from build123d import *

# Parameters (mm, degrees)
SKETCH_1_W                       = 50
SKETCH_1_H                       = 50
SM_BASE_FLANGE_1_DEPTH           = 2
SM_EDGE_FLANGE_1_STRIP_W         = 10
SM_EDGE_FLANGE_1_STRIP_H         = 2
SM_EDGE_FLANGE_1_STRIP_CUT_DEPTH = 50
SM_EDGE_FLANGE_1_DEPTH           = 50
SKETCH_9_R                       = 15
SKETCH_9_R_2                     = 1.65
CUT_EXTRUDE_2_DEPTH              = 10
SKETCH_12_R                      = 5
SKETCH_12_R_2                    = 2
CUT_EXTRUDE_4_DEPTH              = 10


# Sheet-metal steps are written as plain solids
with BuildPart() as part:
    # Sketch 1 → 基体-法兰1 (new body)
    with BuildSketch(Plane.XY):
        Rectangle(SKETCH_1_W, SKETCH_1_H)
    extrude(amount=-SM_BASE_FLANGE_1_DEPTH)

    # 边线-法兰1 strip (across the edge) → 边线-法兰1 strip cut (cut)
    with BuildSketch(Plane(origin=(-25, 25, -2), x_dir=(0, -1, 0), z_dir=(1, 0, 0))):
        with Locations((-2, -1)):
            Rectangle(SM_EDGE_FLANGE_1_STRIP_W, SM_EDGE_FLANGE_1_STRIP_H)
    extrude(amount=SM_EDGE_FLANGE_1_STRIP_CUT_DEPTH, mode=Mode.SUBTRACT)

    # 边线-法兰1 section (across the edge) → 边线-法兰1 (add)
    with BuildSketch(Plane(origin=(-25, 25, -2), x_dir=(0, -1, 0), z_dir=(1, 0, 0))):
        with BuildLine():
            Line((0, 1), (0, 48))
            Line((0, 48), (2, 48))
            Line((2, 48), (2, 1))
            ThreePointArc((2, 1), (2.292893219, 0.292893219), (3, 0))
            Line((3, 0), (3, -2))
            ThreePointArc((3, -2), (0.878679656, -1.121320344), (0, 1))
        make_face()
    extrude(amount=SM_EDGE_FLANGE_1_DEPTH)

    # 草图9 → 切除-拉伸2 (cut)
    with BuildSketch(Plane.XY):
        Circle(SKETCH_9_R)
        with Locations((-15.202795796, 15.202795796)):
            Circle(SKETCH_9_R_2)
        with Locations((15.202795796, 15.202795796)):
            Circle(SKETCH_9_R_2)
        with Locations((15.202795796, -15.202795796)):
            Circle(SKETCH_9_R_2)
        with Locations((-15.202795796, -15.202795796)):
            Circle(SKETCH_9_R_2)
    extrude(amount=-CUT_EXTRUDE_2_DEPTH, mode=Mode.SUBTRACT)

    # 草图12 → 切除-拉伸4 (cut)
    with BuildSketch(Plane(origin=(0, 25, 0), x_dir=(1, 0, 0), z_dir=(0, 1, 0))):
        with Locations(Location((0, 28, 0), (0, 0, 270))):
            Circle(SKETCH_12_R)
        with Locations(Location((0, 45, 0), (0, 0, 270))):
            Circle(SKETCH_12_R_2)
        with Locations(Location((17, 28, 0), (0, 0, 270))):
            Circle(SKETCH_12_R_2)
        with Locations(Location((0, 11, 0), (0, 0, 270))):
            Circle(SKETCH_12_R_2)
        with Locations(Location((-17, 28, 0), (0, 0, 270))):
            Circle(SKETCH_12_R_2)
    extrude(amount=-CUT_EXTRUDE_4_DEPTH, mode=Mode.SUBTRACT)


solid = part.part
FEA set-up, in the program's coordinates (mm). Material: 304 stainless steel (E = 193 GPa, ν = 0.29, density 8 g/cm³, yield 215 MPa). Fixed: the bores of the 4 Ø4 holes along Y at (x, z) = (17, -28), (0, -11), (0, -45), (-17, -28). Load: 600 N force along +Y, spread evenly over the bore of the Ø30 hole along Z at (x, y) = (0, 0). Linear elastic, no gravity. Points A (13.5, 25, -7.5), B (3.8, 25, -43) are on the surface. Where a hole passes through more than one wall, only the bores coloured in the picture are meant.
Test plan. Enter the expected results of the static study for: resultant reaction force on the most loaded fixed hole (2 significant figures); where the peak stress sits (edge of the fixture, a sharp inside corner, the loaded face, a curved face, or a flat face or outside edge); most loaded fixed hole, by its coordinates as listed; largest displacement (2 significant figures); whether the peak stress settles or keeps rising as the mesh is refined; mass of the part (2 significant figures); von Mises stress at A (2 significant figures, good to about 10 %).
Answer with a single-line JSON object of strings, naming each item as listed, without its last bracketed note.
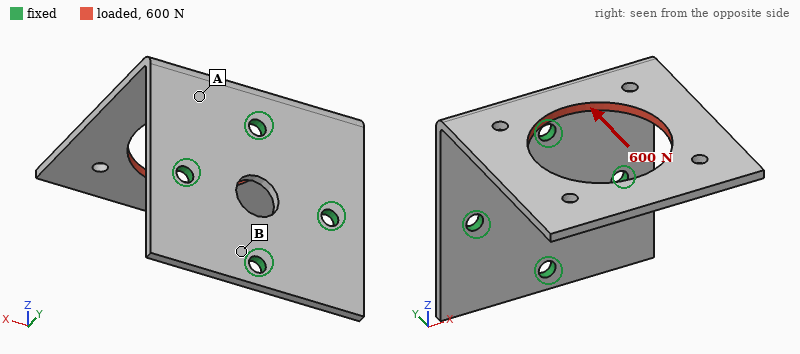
{"resultant reaction force on the most loaded fixed hole": "700 N", "where the peak stress sits": "edge of the fixture", "most loaded fixed hole, by its coordinates as listed": "(0, -11)", "largest displacement": "0.28 mm", "whether the peak stress settles or keeps rising as the mesh is refined": "keeps rising", "mass of the part": "64 g", "von Mises stress at A": "60 MPa"}
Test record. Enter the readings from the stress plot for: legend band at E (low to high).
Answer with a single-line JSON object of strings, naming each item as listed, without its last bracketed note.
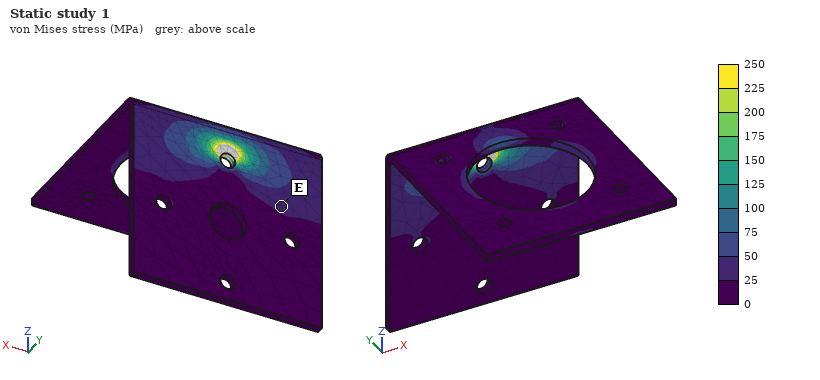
{"legend band at E": "25 to 50 MPa"}
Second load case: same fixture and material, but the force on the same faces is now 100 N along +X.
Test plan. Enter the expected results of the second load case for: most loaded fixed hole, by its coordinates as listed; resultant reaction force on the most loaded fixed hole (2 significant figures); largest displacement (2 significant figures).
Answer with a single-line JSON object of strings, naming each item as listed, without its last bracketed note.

{"most loaded fixed hole, by its coordinates as listed": "(0, -11)", "resultant reaction force on the most loaded fixed hole": "87 N", "largest displacement": "0.12 mm"}
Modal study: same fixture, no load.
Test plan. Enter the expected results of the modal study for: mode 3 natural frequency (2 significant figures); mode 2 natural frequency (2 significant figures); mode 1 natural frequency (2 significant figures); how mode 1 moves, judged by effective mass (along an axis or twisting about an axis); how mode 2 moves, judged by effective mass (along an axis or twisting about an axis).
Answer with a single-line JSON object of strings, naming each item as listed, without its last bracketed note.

{"mode 3 natural frequency": "1300 Hz", "mode 2 natural frequency": "910 Hz", "mode 1 natural frequency": "470 Hz", "how mode 1 moves, judged by effective mass": "along Z", "how mode 2 moves, judged by effective mass": "along X"}
